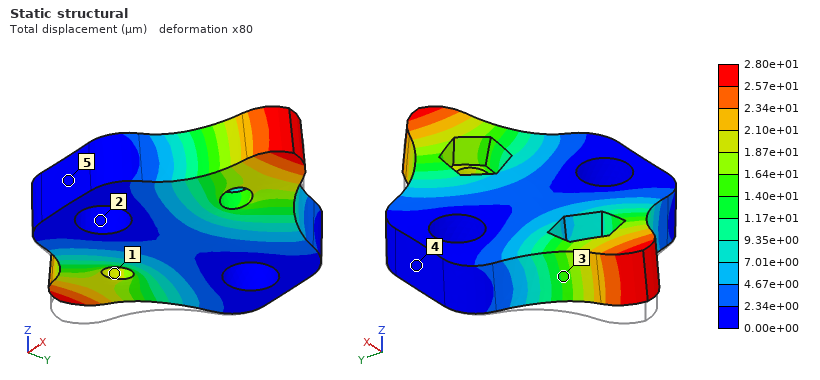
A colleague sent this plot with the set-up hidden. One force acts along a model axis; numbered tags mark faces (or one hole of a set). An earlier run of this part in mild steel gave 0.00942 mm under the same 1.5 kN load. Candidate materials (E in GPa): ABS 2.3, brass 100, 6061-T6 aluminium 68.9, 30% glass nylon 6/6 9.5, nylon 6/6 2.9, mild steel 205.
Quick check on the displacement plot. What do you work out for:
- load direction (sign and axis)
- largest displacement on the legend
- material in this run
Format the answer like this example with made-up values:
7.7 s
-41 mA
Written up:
+Z
2.80e+01 µm
6061-T6 aluminium
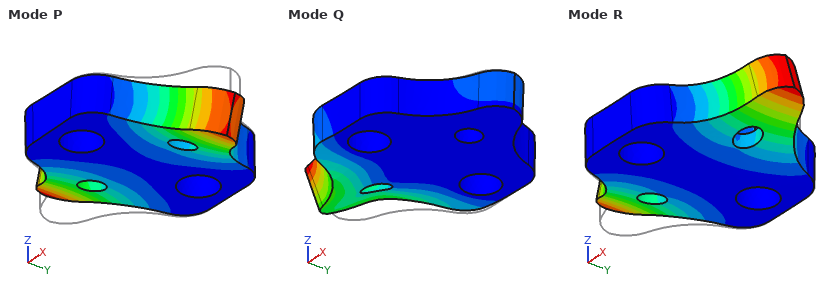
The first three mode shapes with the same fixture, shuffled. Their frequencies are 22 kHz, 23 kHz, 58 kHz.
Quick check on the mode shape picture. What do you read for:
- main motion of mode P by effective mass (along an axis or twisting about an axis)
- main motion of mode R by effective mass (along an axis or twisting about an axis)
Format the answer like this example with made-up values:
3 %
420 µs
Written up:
twisting about Y
along Z
